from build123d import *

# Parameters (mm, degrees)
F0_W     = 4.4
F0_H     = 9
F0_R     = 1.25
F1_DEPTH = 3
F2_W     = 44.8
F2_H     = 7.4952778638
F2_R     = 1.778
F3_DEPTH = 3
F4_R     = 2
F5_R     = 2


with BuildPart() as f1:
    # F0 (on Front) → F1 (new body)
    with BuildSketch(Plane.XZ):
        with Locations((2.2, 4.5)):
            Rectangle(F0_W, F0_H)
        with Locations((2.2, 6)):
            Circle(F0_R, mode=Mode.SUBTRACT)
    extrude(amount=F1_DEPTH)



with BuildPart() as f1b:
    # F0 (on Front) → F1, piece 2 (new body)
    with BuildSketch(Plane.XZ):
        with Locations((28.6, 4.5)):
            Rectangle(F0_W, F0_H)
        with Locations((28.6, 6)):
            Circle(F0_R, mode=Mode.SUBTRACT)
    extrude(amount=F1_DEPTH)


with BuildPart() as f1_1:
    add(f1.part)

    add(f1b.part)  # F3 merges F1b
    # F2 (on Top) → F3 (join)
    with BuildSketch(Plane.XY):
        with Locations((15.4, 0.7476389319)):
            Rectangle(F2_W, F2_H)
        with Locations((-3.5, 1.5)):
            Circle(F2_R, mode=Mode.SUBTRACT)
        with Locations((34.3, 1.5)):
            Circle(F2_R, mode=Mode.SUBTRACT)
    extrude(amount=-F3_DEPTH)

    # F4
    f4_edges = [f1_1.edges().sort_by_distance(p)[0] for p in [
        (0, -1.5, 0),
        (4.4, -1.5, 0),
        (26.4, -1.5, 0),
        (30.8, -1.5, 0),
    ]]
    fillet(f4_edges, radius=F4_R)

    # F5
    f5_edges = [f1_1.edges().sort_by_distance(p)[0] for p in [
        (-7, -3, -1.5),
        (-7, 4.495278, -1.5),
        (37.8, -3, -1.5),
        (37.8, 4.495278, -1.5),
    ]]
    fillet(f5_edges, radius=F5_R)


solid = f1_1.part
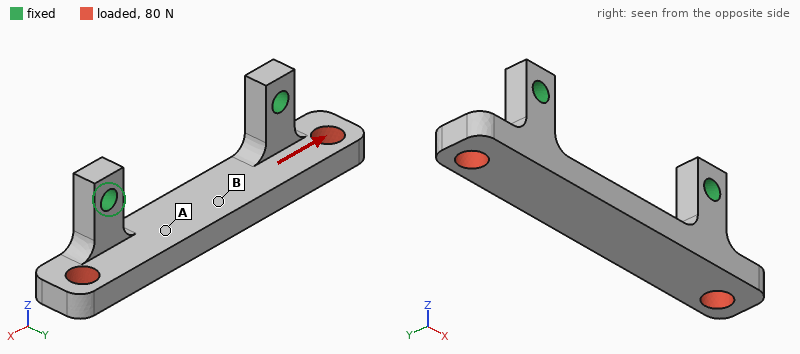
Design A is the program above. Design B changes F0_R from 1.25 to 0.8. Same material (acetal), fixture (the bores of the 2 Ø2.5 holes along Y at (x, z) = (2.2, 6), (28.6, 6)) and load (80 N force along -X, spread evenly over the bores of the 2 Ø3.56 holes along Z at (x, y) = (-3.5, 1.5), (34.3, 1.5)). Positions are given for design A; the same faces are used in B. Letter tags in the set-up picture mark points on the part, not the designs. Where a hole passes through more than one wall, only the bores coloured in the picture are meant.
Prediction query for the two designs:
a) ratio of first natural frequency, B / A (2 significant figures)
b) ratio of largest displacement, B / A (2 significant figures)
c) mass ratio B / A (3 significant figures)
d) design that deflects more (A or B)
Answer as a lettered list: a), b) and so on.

a) 0.91
b) 1.2
c) 1.02
d) B
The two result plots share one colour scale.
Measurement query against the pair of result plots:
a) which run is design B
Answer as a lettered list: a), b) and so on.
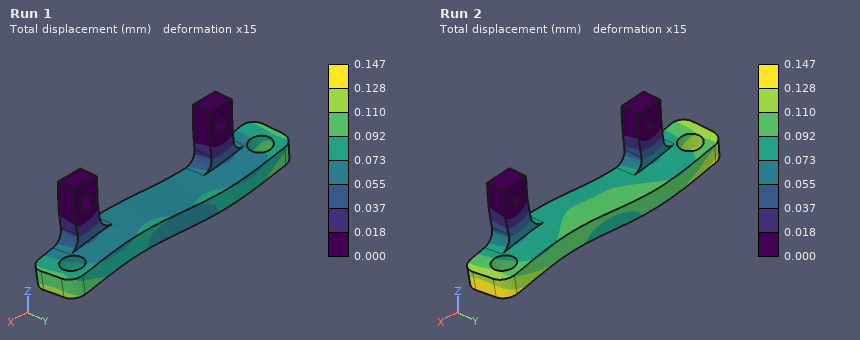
a) Run 2
